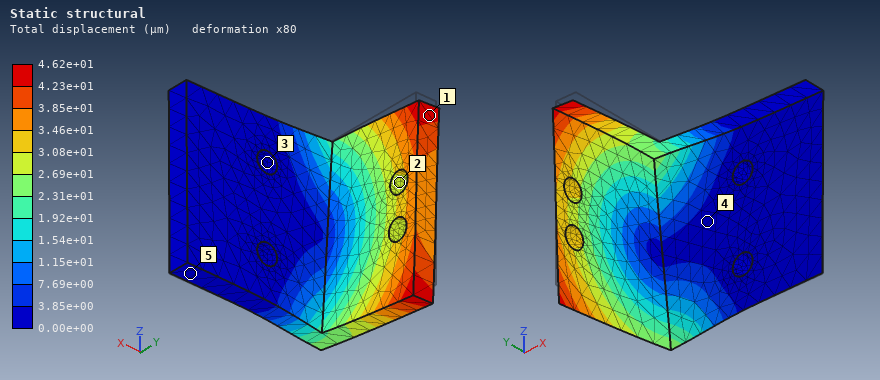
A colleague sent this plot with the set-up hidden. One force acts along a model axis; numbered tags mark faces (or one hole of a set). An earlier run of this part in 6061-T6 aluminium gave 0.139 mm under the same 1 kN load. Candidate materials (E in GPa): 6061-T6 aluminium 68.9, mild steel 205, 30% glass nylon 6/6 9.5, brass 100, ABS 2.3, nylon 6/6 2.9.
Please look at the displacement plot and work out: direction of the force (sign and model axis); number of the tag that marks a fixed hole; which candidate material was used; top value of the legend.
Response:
-Z
3
mild steel
4.62e+01 µm
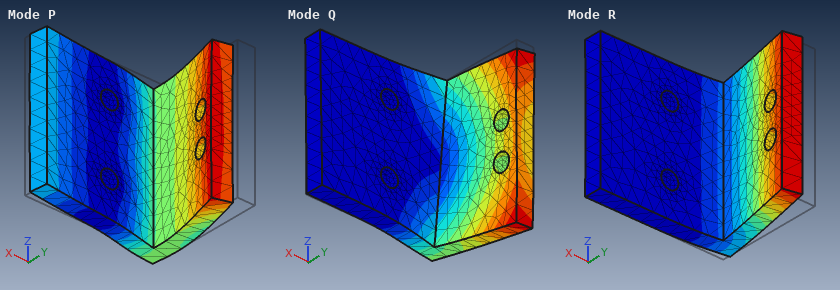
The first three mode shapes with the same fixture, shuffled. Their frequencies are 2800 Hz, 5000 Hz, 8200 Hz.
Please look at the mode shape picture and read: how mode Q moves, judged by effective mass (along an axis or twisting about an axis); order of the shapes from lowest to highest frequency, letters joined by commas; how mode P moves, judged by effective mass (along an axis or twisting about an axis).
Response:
along Z
R, Q, P
along Y
